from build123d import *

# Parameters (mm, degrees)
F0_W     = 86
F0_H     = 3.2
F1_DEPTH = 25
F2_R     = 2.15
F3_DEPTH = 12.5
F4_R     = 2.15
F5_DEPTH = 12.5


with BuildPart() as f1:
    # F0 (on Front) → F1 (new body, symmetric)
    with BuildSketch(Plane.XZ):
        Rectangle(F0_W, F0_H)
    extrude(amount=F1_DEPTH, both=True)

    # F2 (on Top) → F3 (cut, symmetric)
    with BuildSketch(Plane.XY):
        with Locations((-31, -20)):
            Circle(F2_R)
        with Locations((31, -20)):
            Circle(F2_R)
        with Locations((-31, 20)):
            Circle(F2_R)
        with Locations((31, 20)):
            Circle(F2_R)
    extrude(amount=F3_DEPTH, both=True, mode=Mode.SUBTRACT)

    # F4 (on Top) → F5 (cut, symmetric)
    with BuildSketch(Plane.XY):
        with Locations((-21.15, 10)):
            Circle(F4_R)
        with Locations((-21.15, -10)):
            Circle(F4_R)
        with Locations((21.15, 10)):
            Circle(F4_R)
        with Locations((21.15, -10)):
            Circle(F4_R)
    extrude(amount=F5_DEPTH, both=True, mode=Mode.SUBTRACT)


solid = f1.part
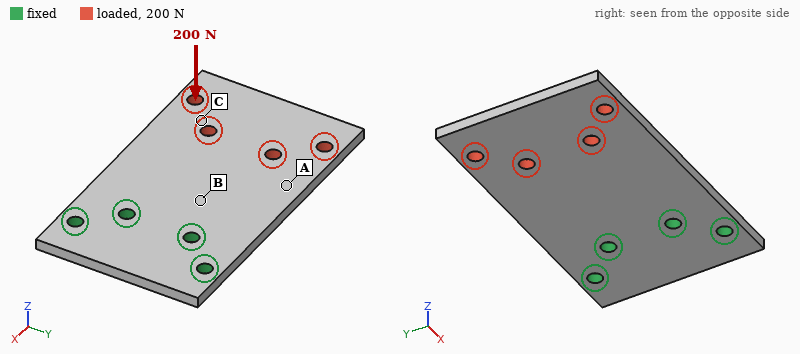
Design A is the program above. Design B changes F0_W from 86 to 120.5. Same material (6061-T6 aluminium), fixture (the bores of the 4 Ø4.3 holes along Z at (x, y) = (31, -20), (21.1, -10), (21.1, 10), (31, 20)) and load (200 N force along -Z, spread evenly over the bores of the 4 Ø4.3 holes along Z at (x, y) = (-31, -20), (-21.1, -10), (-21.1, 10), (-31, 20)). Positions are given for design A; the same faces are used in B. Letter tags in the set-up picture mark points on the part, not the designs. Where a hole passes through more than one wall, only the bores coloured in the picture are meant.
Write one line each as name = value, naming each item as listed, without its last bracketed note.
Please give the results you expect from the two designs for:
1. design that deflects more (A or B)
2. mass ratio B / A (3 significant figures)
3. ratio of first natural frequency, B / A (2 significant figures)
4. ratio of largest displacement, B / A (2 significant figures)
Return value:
design that deflects more = B
mass ratio B / A = 1.41
ratio of first natural frequency, B / A = 0.61
ratio of largest displacement, B / A = 1.4
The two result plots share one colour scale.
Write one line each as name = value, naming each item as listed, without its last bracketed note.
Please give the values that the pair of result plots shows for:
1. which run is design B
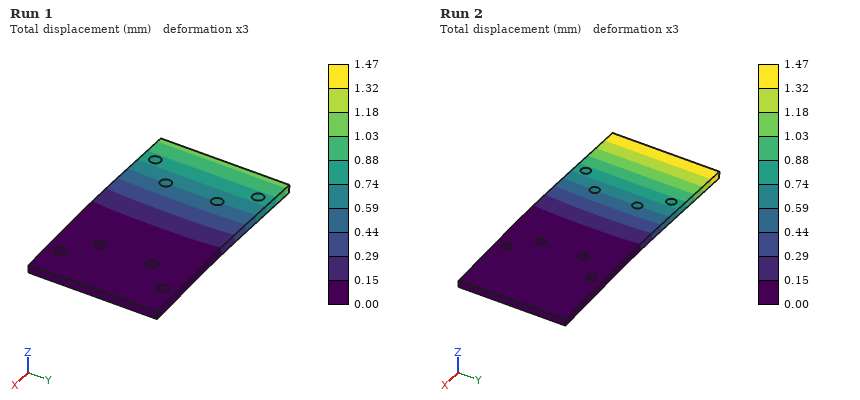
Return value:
which run is design B = Run 2
